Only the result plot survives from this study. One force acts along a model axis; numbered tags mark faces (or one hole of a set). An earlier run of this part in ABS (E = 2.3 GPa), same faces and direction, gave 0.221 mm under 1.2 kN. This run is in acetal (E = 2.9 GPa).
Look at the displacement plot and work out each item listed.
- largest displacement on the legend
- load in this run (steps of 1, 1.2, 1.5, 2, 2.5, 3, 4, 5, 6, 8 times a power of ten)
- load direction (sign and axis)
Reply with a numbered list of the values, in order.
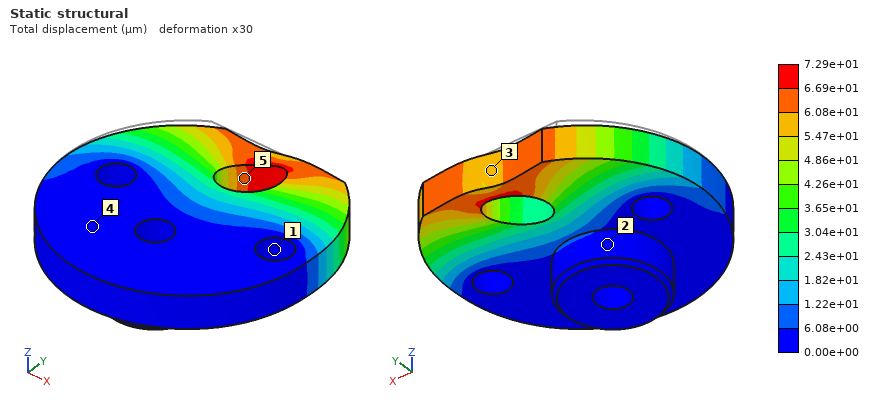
1. 7.29e+01 µm
2. 500 N
3. +X
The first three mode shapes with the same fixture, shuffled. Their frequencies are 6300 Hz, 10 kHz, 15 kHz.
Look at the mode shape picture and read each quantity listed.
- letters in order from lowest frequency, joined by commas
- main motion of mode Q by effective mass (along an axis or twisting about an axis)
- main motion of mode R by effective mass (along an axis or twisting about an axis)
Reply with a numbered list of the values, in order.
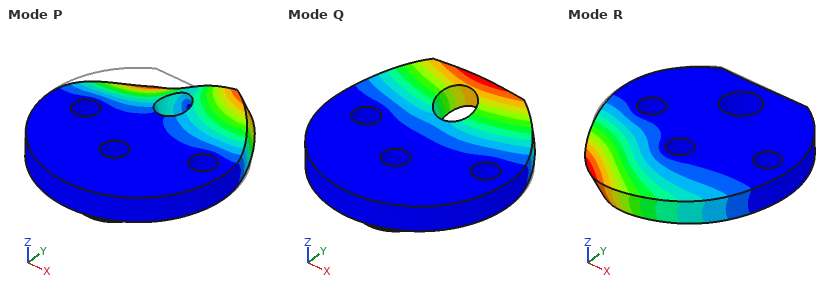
1. Q, P, R
2. along Z
3. along Z
